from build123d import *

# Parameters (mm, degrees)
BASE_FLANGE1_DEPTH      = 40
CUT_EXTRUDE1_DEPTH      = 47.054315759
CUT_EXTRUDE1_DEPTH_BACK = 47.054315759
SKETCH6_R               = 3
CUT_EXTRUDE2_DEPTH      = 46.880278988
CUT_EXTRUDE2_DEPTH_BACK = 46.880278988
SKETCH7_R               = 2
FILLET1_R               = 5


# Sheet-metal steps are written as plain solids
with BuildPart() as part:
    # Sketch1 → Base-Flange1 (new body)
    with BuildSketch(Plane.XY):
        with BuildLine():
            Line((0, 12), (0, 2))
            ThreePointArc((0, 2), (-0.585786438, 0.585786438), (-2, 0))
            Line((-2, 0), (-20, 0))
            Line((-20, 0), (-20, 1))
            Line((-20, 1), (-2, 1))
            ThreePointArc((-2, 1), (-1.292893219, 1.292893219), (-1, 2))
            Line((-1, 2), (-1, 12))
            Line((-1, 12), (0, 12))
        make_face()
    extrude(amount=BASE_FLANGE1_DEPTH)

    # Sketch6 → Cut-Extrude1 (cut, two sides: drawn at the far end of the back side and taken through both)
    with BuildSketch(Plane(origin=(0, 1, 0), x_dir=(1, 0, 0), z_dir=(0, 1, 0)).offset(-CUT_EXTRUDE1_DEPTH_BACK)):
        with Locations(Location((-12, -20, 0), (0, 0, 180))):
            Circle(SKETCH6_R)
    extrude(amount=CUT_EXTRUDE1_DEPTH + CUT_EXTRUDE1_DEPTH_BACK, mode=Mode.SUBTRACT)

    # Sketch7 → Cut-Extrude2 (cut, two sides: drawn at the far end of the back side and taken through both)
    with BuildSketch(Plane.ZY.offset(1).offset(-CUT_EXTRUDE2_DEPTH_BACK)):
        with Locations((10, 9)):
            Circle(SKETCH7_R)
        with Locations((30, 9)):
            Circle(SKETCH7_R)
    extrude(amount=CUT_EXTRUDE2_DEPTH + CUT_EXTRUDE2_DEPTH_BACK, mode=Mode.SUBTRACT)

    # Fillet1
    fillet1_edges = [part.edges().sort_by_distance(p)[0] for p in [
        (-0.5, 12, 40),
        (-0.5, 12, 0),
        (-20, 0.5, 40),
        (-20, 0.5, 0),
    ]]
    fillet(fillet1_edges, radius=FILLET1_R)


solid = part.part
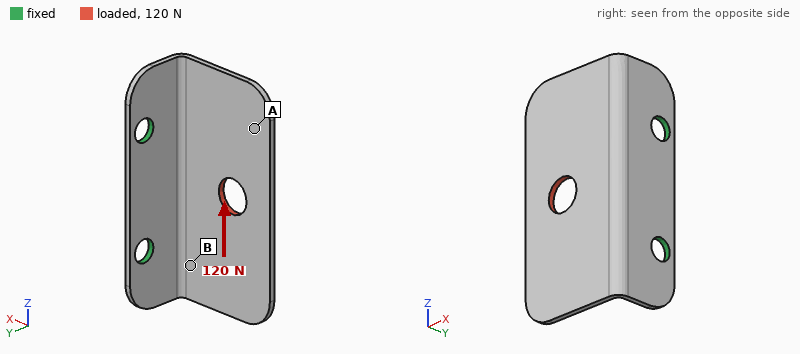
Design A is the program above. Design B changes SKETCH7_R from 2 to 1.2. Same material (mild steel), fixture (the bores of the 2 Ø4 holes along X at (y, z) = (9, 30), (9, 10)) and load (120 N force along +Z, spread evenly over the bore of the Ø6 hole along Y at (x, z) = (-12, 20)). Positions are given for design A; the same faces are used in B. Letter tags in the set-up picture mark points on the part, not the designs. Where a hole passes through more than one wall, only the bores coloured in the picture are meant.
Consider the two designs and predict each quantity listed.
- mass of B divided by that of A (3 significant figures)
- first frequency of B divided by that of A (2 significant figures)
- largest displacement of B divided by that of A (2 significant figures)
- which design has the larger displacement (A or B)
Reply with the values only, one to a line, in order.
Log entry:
1.01
0.93
1.3
B
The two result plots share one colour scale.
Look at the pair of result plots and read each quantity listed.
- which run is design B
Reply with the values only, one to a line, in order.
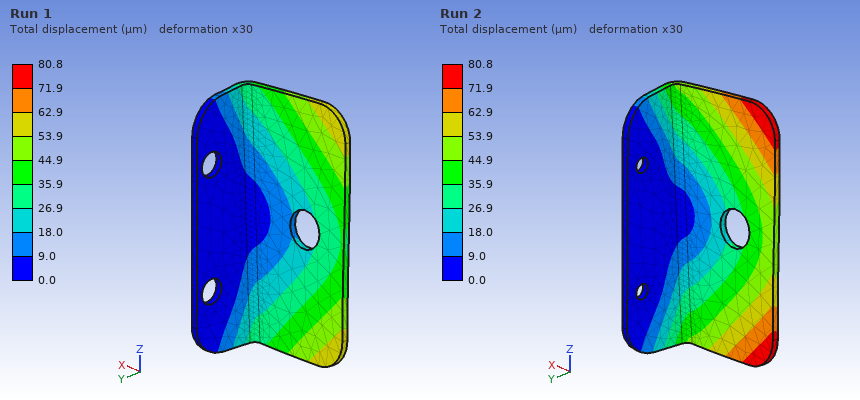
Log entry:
Run 2
